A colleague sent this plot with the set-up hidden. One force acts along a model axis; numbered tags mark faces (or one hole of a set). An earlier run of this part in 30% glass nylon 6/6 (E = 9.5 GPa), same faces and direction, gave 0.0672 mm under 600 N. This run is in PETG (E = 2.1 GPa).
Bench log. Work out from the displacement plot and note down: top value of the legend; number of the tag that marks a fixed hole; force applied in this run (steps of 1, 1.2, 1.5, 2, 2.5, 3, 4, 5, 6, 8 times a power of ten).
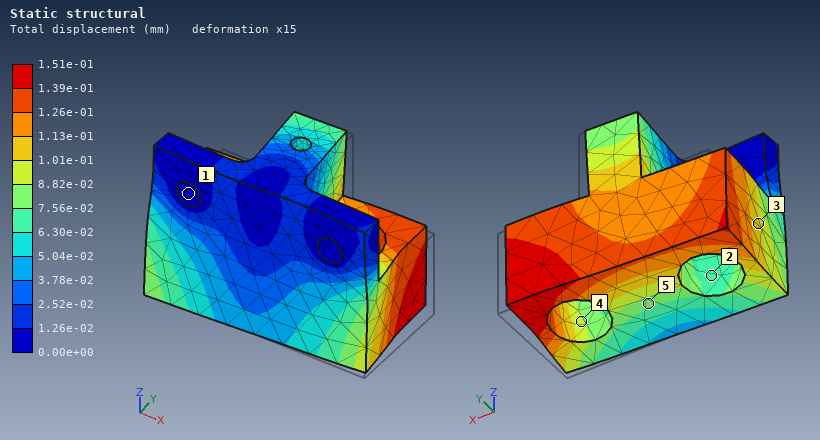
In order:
1.51e-01 mm
1
300 N
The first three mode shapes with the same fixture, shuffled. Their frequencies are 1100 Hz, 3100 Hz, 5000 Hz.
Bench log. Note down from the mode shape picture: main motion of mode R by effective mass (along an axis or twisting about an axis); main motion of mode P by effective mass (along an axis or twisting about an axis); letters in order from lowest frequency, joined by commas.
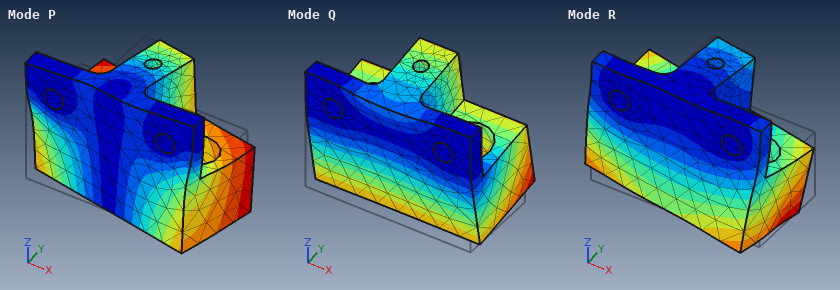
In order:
along X
along X
Q, P, R
